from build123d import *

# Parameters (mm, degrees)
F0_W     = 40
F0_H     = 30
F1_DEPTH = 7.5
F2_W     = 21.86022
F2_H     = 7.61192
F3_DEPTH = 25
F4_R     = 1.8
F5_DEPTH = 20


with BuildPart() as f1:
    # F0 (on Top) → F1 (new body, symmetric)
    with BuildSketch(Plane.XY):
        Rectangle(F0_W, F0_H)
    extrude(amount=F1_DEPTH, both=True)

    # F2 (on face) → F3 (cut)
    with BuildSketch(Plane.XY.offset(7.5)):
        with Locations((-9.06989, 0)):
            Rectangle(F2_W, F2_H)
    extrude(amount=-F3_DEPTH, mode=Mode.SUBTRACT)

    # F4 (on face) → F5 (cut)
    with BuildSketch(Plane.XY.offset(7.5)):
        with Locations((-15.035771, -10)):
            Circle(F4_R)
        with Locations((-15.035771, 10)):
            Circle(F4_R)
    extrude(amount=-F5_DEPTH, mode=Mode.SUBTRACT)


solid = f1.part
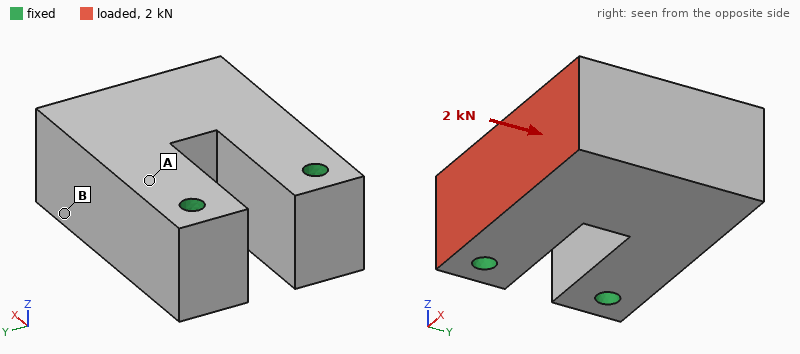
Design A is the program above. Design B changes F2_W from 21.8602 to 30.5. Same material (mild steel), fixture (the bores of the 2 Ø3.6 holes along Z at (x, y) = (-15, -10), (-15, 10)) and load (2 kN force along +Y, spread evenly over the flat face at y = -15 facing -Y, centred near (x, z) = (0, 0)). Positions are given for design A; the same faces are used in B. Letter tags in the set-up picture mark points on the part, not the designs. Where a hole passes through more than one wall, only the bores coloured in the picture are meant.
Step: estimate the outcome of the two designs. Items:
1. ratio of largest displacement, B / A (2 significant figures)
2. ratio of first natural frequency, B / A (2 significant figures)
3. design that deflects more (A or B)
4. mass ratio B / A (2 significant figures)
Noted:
1.2
1.0
B
0.97
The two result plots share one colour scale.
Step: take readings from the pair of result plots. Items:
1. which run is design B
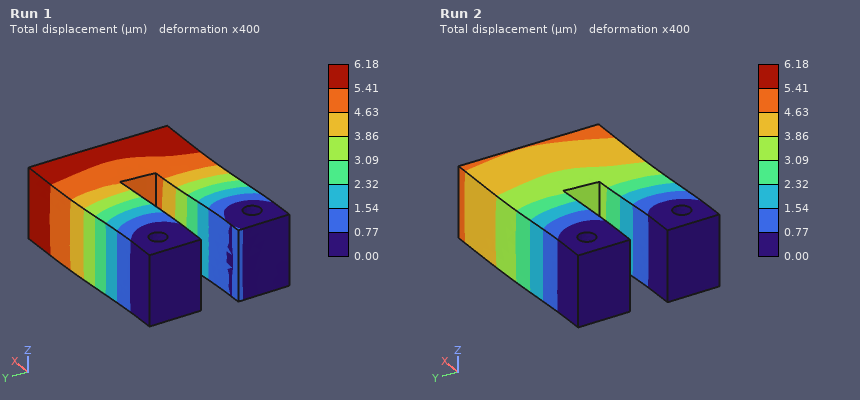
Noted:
Run 1
